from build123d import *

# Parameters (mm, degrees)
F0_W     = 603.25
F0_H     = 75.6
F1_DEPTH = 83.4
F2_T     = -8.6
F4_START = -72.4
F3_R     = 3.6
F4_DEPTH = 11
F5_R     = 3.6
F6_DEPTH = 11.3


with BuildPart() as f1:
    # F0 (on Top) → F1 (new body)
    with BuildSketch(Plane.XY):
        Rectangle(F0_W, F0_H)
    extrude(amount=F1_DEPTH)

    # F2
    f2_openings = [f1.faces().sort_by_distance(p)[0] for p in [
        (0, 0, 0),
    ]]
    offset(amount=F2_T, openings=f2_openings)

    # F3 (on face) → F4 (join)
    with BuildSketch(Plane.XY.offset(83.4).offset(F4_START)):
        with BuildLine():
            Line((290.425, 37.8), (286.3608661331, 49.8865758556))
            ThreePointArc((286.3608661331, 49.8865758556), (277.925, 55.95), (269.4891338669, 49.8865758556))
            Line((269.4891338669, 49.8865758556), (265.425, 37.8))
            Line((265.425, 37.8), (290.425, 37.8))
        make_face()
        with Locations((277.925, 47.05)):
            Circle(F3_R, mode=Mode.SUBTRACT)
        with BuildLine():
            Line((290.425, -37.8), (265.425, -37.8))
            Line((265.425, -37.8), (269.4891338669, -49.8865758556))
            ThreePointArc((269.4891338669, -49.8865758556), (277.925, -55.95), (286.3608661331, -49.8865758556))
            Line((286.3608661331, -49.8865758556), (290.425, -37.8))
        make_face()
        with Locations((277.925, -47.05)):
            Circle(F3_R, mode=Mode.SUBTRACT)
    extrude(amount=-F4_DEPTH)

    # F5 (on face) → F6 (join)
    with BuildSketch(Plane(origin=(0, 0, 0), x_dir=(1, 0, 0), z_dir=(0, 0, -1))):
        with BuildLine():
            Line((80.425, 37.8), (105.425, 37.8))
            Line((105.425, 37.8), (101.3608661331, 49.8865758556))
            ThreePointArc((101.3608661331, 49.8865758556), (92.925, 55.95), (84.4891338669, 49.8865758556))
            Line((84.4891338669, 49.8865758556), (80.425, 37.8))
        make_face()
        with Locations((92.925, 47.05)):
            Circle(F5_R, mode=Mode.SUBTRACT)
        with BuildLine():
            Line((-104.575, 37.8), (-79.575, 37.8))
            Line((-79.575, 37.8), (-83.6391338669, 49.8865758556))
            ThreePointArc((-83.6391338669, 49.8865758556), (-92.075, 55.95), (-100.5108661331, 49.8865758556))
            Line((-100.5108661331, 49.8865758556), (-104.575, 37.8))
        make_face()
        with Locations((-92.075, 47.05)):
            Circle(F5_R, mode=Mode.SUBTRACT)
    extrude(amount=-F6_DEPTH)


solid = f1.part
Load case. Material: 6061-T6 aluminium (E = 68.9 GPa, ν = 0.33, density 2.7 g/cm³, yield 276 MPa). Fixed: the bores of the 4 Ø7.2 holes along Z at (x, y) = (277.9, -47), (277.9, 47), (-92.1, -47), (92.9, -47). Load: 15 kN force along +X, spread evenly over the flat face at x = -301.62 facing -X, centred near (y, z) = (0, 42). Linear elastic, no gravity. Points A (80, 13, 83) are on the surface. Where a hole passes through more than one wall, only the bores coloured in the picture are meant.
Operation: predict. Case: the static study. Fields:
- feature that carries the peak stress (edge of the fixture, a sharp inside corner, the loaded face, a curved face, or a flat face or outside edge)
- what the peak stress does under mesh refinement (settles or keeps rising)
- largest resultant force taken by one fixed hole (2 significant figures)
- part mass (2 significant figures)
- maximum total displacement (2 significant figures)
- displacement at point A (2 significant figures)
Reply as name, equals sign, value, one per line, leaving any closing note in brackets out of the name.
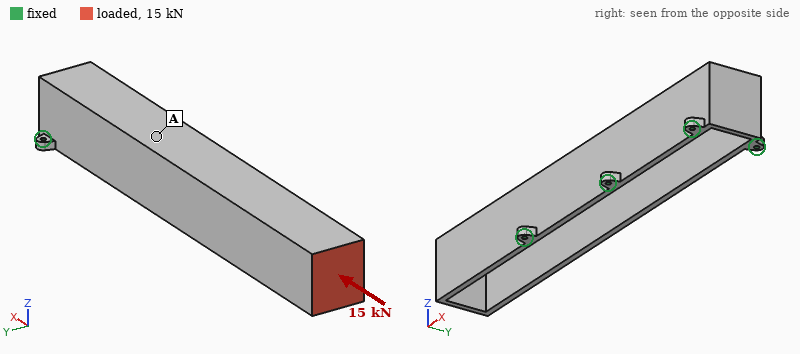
feature that carries the peak stress = edge of the fixture
what the peak stress does under mesh refinement = keeps rising
largest resultant force taken by one fixed hole = 5.1 kN
part mass = 3.4 kg
maximum total displacement = 0.26 mm
displacement at point A = 0.053 mm
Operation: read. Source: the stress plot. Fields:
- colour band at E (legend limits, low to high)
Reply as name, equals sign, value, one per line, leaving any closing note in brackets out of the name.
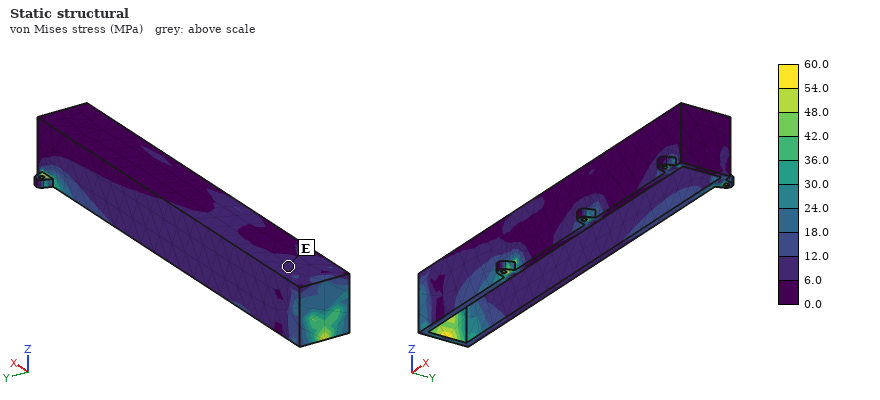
colour band at E = 6.0 to 12.0 MPa
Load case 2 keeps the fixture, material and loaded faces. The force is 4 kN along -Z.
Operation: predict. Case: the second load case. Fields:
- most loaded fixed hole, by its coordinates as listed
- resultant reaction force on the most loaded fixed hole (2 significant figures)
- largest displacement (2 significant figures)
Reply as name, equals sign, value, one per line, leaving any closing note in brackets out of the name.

most loaded fixed hole, by its coordinates as listed = (-92.1, -47)
resultant reaction force on the most loaded fixed hole = 7.3 kN
largest displacement = 1.2 mm
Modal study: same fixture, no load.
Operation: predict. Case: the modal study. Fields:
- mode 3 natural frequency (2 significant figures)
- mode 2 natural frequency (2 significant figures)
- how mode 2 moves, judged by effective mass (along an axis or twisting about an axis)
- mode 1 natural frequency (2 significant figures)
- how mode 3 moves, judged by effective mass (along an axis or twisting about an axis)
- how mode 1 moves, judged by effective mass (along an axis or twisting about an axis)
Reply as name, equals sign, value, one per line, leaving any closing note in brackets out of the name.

mode 3 natural frequency = 590 Hz
mode 2 natural frequency = 330 Hz
how mode 2 moves, judged by effective mass = along Z
mode 1 natural frequency = 280 Hz
how mode 3 moves, judged by effective mass = along Y
how mode 1 moves, judged by effective mass = along Y
